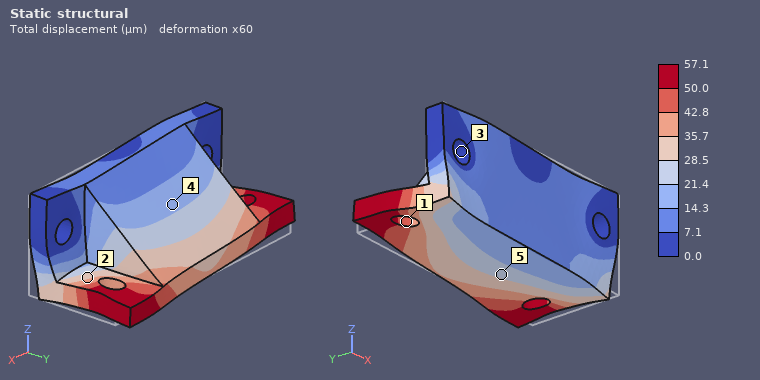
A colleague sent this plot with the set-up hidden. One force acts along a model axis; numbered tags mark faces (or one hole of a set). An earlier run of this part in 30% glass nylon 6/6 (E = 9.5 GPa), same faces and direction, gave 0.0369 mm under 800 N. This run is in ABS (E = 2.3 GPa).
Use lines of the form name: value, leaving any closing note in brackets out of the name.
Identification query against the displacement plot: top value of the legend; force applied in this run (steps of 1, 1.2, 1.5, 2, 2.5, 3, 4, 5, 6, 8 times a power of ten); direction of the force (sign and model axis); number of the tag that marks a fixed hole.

top value of the legend: 57.1 µm
force applied in this run: 300 N
direction of the force: -X
number of the tag that marks a fixed hole: 3
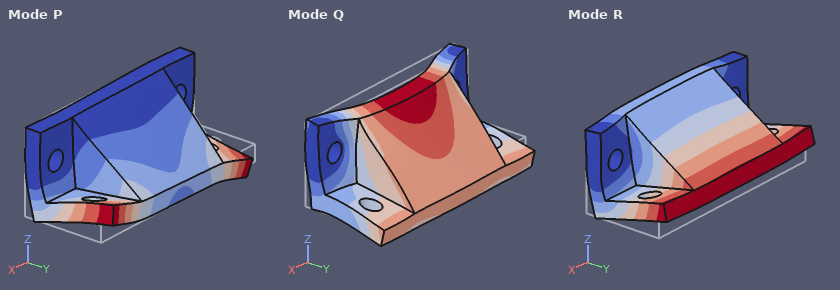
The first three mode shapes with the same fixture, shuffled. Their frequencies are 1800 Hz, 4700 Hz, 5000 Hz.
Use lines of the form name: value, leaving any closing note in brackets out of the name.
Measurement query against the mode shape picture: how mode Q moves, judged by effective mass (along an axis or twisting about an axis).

how mode Q moves, judged by effective mass: along Y
